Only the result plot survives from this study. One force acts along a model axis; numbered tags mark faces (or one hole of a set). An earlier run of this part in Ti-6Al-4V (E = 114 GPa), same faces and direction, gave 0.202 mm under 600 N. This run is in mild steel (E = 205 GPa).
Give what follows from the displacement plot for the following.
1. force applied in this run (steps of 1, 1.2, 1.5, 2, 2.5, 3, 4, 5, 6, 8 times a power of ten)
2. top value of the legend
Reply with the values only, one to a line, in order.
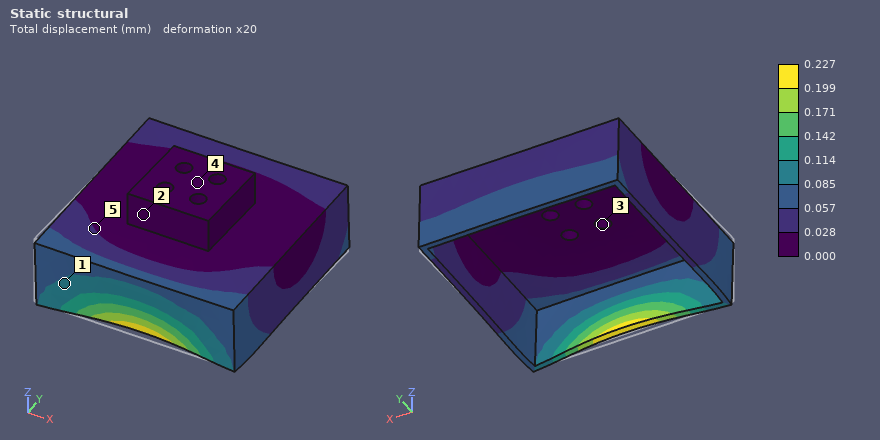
1.2 kN
0.227 mm
